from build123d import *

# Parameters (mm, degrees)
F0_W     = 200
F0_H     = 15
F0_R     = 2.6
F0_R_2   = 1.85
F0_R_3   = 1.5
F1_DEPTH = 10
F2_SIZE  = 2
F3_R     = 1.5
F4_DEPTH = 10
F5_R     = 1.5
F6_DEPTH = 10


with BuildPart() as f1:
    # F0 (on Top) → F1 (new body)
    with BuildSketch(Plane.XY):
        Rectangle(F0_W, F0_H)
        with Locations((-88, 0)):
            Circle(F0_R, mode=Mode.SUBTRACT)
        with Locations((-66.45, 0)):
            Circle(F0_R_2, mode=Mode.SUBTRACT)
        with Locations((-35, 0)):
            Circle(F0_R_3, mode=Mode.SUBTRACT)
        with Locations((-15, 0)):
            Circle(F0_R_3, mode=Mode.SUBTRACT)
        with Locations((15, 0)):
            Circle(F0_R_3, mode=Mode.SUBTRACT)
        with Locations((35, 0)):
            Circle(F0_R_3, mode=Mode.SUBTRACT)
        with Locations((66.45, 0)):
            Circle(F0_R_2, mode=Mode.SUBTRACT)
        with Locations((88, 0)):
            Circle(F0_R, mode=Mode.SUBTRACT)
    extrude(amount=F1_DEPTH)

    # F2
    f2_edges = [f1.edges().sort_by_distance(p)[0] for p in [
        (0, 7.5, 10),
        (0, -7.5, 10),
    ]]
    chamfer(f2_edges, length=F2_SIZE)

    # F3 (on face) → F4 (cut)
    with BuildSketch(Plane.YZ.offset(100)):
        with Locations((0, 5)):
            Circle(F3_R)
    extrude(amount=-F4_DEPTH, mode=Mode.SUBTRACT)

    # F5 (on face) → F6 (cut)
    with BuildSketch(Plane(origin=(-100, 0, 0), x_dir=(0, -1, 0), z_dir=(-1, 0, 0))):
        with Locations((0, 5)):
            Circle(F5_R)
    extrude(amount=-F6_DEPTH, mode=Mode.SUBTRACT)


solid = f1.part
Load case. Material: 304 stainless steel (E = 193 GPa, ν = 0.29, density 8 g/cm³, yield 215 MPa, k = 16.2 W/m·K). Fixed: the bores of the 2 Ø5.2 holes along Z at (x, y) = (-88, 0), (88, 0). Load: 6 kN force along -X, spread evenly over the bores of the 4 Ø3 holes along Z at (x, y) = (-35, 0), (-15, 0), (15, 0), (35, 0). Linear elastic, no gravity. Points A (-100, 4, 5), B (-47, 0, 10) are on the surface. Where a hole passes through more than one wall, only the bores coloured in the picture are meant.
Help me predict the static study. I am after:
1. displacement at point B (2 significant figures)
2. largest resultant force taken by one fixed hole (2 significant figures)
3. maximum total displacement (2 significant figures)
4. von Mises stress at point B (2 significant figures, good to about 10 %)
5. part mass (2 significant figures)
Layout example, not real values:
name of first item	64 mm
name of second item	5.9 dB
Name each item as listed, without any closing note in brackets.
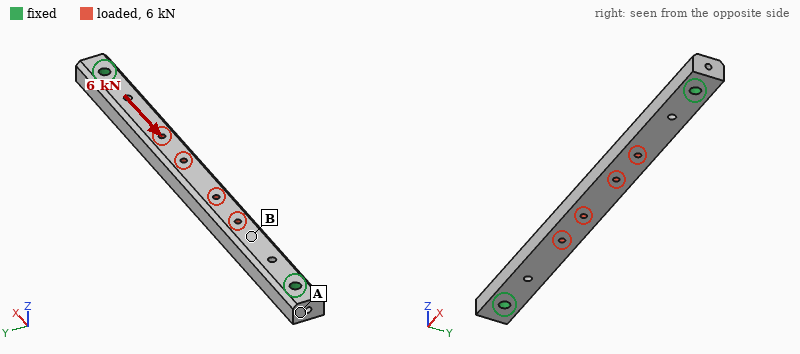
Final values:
displacement at point B	4.6 µm
largest resultant force taken by one fixed hole	3.0 kN
maximum total displacement	7.5 µm
von Mises stress at point B	21 MPa
part mass	230 g
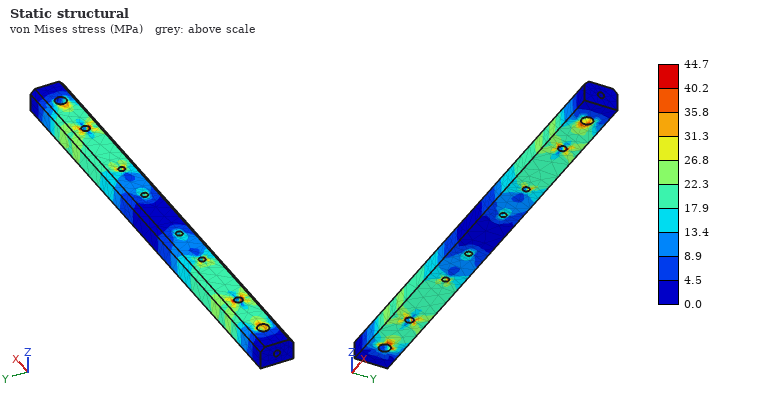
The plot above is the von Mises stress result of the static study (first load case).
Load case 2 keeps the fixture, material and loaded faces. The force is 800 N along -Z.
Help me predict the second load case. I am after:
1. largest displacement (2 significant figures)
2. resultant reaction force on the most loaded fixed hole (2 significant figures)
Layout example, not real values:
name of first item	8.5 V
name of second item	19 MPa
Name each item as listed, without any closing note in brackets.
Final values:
largest displacement	83 µm
resultant reaction force on the most loaded fixed hole	400 N
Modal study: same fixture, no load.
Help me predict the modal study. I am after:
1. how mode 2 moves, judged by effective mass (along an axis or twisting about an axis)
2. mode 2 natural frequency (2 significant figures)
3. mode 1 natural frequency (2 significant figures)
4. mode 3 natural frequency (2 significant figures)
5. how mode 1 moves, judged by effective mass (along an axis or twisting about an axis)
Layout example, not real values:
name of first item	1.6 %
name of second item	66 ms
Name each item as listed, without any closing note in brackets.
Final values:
how mode 2 moves, judged by effective mass	along Y
mode 2 natural frequency	2100 Hz
mode 1 natural frequency	1600 Hz
mode 3 natural frequency	4300 Hz
how mode 1 moves, judged by effective mass	along Z
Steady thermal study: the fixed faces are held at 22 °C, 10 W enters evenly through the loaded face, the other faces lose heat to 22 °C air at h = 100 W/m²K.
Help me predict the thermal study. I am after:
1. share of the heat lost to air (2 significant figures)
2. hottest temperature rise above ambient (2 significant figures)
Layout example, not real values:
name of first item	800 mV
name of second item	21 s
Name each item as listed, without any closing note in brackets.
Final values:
share of the heat lost to air	93 %
hottest temperature rise above ambient	23 K
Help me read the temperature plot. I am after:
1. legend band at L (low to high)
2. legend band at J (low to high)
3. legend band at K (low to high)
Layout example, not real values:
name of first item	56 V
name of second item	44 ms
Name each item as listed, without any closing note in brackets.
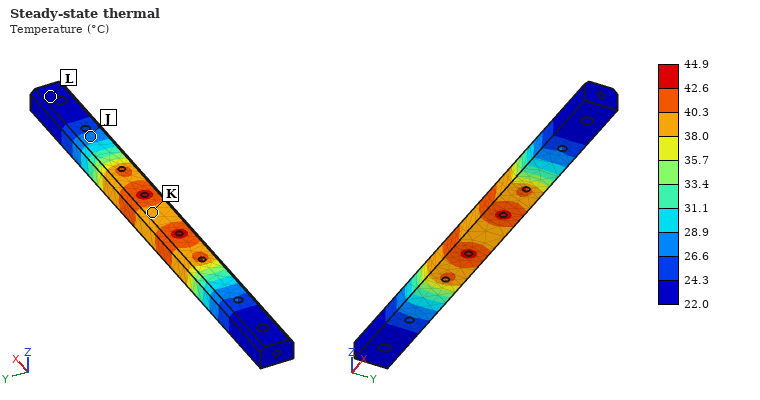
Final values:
legend band at L	22.0 to 24.3 °C
legend band at J	26.6 to 28.9 °C
legend band at K	38.0 to 40.3 °C
